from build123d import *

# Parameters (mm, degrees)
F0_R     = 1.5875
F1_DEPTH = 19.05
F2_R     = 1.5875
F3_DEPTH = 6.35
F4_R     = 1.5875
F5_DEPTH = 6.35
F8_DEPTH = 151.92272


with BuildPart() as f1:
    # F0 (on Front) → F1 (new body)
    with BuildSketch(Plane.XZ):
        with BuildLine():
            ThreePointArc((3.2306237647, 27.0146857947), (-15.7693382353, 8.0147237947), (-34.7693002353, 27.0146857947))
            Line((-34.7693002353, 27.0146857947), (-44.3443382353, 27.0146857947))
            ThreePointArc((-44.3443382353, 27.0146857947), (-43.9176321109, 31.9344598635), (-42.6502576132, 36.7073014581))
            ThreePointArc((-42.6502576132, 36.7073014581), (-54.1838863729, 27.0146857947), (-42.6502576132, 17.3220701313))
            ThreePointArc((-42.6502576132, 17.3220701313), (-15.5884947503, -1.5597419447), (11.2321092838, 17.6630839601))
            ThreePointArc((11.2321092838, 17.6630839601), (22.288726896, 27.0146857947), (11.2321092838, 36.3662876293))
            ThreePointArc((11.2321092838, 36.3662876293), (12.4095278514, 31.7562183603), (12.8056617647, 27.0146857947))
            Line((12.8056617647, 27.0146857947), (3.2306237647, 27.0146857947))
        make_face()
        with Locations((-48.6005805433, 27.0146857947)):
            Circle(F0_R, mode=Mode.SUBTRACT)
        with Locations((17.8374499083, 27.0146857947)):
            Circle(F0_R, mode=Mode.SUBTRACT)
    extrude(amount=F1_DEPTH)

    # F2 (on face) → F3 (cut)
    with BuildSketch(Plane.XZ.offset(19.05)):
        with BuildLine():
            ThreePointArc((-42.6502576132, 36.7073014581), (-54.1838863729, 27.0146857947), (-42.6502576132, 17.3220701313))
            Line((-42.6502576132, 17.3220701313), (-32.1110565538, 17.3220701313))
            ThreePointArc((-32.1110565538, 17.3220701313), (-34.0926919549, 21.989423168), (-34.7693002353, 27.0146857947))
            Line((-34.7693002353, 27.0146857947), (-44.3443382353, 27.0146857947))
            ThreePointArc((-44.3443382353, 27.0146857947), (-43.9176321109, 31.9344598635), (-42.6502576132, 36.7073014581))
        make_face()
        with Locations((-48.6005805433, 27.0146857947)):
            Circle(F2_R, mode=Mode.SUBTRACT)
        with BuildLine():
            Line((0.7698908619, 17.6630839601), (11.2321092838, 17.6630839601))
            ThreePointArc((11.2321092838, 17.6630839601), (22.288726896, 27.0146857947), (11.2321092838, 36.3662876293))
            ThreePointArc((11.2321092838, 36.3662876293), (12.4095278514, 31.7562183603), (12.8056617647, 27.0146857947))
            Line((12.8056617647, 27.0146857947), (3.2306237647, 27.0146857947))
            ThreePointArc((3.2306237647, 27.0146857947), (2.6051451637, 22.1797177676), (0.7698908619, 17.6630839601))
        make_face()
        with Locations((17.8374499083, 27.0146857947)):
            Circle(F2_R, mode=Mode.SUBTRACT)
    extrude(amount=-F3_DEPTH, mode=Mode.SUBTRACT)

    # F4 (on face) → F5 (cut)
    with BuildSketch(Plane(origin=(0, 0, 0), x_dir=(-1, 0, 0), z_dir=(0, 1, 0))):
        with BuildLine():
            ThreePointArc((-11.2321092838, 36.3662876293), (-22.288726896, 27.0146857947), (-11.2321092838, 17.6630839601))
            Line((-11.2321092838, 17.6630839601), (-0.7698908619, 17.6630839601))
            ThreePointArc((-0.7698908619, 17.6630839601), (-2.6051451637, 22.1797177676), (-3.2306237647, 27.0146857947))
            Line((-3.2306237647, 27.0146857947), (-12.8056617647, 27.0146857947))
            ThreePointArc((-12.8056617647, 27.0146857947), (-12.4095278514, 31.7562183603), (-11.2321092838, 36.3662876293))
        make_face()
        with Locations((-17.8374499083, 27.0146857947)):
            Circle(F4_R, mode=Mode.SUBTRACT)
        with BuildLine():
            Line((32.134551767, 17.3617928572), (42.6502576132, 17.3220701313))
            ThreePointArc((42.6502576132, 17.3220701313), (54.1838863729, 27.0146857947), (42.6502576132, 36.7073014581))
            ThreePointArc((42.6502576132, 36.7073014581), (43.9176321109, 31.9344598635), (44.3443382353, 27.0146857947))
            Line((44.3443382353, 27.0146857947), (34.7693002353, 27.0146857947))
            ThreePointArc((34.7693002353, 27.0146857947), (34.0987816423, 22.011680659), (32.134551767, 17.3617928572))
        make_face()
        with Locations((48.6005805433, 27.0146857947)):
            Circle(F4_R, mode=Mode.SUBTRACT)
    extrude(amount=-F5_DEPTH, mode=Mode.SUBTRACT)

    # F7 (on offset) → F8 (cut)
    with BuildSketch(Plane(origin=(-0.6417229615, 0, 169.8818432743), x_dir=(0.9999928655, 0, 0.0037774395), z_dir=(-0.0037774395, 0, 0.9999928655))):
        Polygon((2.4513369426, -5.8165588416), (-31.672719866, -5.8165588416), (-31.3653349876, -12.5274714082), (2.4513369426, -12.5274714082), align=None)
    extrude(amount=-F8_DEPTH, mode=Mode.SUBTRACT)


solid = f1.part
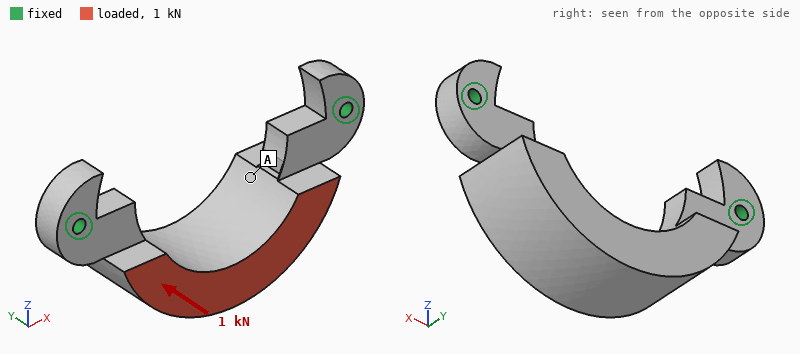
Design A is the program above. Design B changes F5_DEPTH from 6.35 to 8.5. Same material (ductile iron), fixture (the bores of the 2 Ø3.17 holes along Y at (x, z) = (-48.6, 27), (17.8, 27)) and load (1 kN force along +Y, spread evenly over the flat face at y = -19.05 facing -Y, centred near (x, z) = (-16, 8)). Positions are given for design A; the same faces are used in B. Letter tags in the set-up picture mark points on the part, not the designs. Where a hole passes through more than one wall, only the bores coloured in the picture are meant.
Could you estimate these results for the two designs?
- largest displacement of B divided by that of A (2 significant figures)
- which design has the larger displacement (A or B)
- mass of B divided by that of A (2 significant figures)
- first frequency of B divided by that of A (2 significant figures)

2.7
B
0.92
0.61
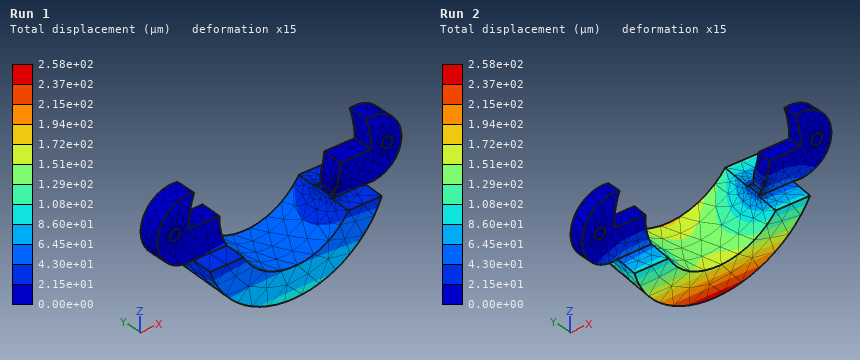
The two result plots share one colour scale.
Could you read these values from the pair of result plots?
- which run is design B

Run 2
